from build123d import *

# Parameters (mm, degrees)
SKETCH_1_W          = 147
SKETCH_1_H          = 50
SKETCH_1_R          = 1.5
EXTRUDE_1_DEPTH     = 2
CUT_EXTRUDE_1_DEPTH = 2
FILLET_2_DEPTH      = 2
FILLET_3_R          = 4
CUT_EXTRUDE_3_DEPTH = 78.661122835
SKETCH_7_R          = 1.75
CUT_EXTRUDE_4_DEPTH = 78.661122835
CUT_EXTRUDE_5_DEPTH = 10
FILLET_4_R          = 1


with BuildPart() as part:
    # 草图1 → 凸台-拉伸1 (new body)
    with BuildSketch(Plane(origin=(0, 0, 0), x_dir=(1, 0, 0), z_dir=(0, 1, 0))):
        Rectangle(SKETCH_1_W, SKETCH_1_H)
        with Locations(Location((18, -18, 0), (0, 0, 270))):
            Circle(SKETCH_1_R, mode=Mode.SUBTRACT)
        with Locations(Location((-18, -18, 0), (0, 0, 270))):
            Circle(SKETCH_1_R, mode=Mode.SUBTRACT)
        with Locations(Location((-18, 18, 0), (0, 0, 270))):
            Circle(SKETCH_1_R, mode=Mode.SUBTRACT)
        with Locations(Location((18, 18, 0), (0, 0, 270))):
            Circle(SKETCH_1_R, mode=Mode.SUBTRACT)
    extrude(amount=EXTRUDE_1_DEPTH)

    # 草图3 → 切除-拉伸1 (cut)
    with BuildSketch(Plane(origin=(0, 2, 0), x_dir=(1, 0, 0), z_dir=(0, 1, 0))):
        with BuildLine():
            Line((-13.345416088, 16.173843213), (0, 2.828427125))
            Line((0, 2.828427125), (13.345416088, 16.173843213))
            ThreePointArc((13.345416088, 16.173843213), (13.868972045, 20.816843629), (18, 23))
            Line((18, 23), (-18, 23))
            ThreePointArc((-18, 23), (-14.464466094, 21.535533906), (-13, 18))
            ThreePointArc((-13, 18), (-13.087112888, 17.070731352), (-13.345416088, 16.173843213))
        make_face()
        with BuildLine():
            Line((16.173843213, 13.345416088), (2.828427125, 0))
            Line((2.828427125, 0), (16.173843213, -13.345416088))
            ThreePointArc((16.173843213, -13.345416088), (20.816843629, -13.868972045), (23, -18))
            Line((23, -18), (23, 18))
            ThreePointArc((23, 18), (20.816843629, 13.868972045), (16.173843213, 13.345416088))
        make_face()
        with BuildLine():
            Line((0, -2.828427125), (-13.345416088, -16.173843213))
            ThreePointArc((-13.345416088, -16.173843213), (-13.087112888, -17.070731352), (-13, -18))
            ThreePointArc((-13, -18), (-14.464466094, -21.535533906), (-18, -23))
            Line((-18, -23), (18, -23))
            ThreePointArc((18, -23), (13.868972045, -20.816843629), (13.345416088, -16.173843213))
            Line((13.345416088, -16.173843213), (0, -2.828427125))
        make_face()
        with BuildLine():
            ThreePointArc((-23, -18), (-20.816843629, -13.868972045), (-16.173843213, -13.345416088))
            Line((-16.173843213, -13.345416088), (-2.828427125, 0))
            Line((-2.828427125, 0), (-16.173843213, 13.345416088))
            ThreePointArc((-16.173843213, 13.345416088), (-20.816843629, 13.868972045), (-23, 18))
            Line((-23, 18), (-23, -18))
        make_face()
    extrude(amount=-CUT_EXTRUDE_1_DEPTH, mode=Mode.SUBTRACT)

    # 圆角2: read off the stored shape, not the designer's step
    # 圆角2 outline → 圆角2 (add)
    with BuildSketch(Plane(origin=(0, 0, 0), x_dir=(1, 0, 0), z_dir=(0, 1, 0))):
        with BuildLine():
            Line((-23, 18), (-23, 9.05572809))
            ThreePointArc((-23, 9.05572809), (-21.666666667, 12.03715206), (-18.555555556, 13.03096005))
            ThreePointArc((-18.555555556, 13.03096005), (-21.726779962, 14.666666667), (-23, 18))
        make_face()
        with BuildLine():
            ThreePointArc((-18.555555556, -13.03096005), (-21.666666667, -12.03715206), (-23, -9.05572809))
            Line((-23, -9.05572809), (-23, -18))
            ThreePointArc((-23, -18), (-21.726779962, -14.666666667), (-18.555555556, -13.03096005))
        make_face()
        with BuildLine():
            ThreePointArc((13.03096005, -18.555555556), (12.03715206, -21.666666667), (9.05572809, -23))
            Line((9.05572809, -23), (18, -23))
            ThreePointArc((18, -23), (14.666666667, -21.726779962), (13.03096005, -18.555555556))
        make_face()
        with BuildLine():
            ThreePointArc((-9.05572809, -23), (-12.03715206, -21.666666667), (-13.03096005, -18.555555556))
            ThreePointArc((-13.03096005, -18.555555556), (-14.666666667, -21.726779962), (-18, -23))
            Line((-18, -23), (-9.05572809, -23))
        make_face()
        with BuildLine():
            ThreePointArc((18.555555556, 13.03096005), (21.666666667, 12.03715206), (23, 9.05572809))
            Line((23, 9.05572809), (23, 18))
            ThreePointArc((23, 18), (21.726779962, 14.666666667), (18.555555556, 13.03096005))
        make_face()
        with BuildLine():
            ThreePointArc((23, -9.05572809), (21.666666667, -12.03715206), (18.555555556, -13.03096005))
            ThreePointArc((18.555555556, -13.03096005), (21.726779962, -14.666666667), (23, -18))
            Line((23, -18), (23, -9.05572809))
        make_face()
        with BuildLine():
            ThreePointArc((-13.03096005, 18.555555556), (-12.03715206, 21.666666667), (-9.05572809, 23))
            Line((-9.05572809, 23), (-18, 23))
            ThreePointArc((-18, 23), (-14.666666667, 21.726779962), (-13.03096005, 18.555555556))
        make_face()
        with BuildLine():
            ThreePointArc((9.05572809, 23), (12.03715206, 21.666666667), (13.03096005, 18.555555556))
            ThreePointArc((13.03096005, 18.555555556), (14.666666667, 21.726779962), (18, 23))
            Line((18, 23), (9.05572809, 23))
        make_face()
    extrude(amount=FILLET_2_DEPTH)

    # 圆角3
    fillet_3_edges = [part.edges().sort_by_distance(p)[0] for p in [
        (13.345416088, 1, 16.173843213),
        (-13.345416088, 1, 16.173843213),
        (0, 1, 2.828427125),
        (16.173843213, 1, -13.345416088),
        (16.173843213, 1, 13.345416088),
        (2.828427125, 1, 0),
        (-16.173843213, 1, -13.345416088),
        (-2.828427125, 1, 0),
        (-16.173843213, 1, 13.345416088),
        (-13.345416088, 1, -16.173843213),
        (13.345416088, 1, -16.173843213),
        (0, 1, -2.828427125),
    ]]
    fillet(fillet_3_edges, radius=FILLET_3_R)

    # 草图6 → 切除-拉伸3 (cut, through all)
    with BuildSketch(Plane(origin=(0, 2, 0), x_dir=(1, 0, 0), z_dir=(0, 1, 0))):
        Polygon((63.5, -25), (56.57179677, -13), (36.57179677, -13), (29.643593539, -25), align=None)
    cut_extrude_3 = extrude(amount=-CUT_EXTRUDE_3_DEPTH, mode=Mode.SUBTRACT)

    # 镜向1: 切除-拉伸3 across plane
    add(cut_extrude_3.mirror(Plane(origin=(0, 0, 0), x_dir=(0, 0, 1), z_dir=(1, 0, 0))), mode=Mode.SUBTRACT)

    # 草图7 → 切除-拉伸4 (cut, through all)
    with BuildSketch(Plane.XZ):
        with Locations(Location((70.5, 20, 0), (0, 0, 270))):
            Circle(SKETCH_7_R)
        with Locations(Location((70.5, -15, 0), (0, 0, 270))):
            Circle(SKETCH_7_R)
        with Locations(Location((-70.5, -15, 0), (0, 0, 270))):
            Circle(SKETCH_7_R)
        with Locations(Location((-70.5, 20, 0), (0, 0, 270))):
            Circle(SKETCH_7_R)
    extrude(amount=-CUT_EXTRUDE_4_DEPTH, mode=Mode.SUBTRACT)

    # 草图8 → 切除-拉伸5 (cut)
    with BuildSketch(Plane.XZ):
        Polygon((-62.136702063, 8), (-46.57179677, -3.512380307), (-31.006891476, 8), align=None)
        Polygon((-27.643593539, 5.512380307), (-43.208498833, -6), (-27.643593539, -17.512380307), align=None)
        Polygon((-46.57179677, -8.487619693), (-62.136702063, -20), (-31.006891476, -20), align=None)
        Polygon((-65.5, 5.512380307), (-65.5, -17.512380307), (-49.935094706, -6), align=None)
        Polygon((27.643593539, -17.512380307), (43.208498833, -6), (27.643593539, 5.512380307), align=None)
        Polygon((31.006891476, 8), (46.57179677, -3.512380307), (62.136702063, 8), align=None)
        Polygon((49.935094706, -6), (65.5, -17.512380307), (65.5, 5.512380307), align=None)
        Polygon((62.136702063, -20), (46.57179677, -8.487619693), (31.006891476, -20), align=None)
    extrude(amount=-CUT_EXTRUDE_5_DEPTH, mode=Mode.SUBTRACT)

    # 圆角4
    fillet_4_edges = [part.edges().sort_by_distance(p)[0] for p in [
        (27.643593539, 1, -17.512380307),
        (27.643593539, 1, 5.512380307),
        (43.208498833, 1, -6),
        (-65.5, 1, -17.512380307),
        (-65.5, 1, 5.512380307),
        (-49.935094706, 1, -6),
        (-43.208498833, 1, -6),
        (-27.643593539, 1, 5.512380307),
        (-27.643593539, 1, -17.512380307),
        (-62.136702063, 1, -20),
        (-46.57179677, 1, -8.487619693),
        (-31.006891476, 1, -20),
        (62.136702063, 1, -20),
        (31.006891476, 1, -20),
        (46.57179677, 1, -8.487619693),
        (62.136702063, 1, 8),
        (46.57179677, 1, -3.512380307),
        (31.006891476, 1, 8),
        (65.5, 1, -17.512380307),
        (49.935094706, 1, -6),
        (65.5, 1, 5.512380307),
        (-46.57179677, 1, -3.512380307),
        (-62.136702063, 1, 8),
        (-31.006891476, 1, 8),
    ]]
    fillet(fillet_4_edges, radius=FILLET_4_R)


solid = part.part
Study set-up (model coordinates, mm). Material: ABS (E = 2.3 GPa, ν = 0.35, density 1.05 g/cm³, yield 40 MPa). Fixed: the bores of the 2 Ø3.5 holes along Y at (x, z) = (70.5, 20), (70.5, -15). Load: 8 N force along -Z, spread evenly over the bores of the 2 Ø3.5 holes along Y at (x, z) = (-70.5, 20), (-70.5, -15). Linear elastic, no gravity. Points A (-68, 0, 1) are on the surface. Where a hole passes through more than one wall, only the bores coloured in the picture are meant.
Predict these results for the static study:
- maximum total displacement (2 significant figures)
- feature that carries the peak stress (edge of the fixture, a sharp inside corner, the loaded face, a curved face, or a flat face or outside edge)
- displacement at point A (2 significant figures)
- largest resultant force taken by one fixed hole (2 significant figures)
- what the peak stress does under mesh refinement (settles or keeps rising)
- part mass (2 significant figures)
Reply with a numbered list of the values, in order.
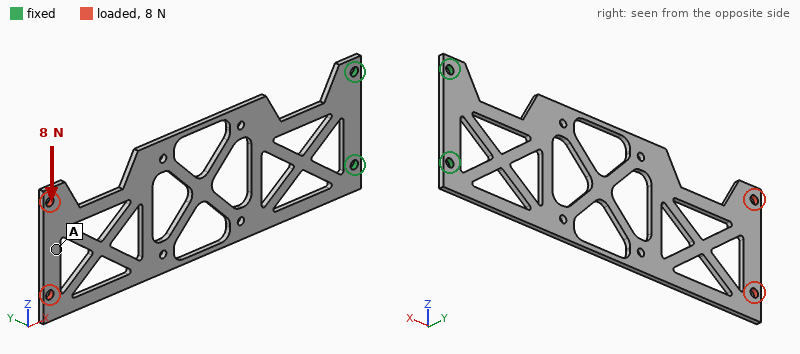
1. 1.0 mm
2. edge of the fixture
3. 0.94 mm
4. 32 N
5. keeps rising
6. 8.1 g
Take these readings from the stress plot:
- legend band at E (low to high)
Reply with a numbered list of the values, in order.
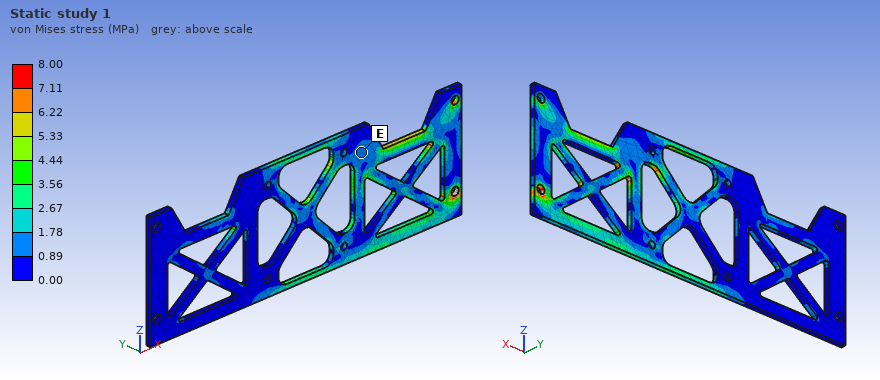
1. 0.89 to 1.78 MPa
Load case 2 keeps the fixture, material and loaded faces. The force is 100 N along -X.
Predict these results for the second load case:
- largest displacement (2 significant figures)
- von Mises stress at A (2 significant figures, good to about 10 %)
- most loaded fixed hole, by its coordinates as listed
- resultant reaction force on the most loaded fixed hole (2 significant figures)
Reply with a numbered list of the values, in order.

1. 1.7 mm
2. 4.8 MPa
3. (70.5, 20)
4. 58 N
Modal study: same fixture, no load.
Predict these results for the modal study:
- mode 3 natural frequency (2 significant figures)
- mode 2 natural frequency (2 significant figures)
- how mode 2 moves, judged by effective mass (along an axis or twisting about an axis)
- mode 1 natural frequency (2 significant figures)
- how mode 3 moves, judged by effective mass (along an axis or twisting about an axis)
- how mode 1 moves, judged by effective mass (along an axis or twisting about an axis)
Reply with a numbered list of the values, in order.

1. 110 Hz
2. 100 Hz
3. twisting about X
4. 18 Hz
5. along Y
6. along Y
